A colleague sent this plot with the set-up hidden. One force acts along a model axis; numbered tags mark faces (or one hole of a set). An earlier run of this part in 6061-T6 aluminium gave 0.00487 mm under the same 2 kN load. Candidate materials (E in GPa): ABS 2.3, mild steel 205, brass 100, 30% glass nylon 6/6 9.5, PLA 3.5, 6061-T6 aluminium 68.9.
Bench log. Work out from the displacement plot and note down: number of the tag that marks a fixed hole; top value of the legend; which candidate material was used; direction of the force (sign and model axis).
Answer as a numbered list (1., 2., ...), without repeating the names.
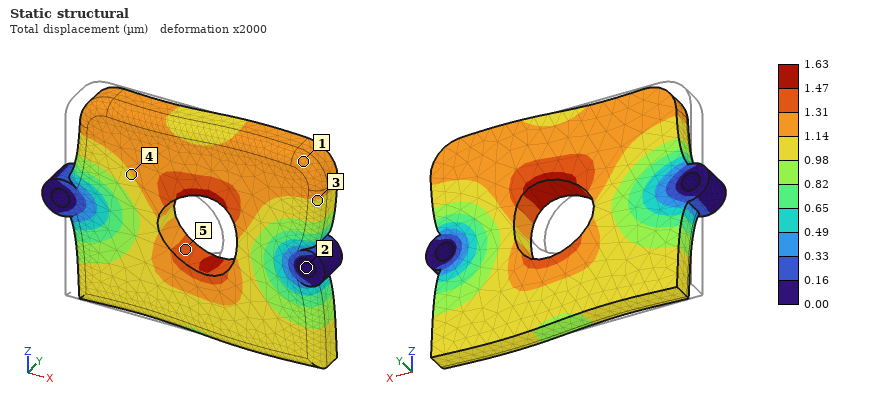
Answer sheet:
1. 2
2. 1.63 µm
3. mild steel
4. +X
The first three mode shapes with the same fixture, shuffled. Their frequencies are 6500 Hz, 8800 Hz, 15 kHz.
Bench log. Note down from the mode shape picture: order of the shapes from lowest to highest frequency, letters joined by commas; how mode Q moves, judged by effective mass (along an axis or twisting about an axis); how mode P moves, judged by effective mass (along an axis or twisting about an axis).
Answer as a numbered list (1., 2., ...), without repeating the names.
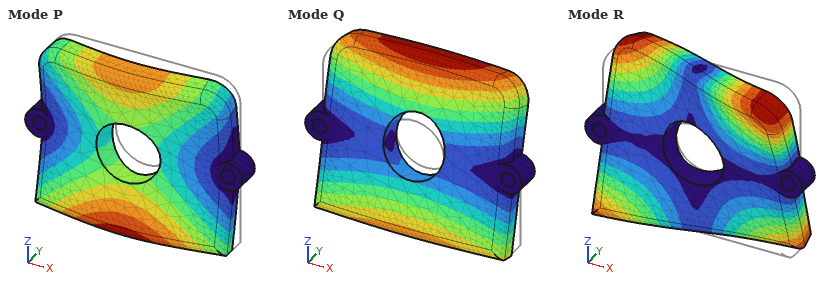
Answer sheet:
1. Q, P, R
2. twisting about X
3. along Y
